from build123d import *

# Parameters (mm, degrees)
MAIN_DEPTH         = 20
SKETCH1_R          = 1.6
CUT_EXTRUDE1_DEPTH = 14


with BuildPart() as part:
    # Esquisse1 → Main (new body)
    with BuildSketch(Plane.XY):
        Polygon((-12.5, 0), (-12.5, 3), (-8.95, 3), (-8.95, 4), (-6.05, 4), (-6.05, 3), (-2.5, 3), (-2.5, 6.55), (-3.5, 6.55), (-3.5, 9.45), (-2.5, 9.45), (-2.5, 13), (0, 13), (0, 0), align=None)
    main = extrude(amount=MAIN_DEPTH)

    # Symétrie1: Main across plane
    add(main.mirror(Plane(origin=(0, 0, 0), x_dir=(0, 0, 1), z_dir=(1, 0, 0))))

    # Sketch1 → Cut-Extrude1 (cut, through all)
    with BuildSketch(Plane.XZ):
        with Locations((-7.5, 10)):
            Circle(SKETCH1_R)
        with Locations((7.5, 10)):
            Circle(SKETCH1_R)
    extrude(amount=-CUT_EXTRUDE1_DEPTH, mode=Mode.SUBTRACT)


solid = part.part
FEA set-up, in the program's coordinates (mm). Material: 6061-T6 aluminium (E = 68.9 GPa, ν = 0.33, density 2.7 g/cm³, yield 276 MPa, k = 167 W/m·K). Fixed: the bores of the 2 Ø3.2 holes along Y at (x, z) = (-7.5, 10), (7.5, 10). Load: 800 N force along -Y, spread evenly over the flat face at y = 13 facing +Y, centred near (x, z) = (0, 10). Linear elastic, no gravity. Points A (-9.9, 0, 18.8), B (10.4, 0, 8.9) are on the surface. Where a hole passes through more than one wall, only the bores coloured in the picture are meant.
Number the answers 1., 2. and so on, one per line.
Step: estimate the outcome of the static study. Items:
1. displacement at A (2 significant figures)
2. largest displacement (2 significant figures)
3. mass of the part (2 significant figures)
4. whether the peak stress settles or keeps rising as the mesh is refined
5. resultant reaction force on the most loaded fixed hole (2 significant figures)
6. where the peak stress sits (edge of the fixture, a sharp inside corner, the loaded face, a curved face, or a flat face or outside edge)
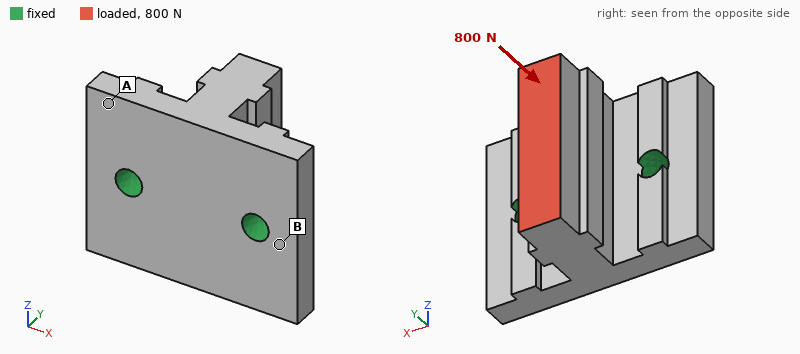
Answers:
1. 2.0 µm
2. 7.0 µm
3. 7.2 g
4. keeps rising
5. 410 N
6. edge of the fixture
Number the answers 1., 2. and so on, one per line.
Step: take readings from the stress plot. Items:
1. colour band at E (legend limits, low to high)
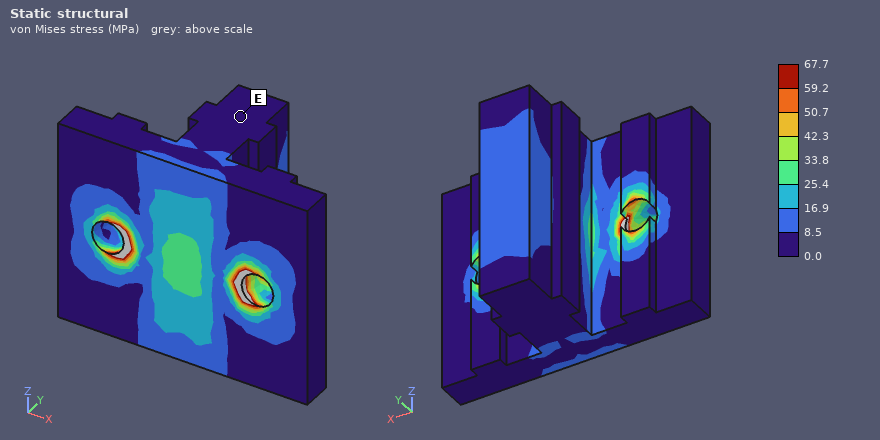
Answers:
1. 0.0 to 8.5 MPa
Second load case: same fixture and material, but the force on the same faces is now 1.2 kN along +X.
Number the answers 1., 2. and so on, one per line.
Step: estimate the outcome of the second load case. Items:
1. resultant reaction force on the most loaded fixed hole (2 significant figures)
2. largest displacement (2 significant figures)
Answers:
1. 1.3 kN
2. 73 µm
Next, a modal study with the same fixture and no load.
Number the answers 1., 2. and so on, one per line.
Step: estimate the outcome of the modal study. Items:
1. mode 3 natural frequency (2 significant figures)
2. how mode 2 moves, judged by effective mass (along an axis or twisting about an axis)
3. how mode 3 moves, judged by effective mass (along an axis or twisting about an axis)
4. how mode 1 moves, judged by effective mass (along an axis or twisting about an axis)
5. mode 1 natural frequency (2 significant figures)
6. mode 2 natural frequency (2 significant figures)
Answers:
1. 27 kHz
2. along X
3. along Y
4. along Z
5. 14 kHz
6. 20 kHz
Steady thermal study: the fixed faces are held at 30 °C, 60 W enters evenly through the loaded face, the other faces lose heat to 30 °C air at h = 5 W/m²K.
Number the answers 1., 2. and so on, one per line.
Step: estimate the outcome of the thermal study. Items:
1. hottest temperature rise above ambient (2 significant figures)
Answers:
1. 59 K
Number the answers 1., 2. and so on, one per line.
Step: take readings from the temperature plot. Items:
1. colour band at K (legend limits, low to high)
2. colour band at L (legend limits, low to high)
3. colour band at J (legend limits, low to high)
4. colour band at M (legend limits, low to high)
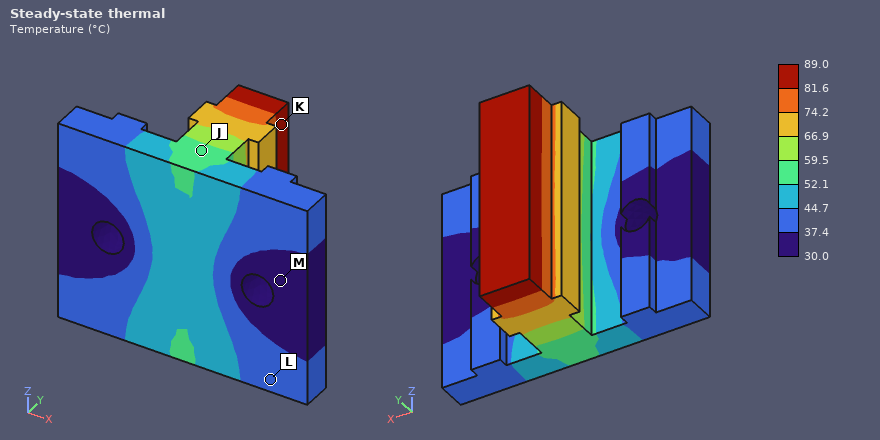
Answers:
1. 81.6 to 89.0 °C
2. 37.4 to 44.7 °C
3. 52.1 to 59.5 °C
4. 30.0 to 37.4 °C
